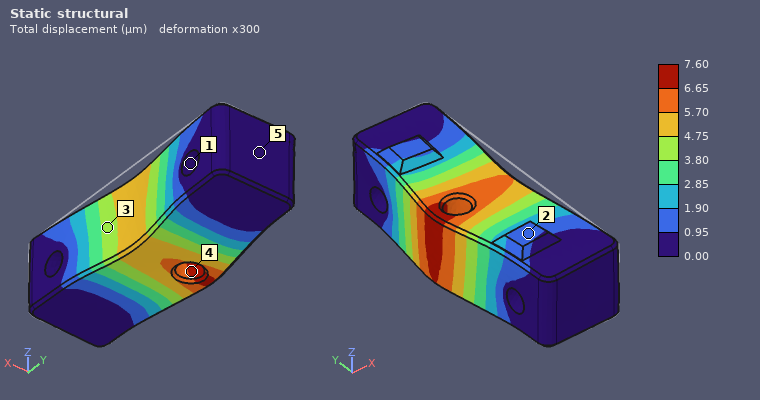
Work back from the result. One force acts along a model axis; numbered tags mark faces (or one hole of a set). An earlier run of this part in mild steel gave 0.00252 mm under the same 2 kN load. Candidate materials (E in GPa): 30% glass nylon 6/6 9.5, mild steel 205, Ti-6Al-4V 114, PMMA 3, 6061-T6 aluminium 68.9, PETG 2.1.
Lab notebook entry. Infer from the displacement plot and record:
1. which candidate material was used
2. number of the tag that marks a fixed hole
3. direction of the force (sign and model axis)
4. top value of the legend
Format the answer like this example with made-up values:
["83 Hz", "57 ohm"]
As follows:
["6061-T6 aluminium", "1", "-X", "7.60 µm"]
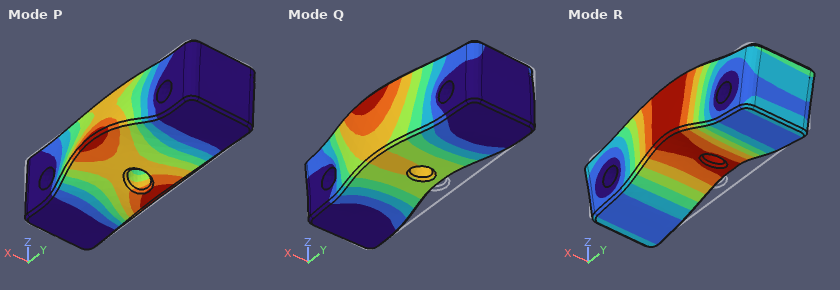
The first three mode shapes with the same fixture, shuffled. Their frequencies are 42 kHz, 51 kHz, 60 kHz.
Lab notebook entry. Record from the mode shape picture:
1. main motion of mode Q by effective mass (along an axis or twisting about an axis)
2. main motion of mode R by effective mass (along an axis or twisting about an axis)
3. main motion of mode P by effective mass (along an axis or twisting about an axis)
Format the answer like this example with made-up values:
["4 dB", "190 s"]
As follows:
["along X", "along Z", "twisting about Y"]
